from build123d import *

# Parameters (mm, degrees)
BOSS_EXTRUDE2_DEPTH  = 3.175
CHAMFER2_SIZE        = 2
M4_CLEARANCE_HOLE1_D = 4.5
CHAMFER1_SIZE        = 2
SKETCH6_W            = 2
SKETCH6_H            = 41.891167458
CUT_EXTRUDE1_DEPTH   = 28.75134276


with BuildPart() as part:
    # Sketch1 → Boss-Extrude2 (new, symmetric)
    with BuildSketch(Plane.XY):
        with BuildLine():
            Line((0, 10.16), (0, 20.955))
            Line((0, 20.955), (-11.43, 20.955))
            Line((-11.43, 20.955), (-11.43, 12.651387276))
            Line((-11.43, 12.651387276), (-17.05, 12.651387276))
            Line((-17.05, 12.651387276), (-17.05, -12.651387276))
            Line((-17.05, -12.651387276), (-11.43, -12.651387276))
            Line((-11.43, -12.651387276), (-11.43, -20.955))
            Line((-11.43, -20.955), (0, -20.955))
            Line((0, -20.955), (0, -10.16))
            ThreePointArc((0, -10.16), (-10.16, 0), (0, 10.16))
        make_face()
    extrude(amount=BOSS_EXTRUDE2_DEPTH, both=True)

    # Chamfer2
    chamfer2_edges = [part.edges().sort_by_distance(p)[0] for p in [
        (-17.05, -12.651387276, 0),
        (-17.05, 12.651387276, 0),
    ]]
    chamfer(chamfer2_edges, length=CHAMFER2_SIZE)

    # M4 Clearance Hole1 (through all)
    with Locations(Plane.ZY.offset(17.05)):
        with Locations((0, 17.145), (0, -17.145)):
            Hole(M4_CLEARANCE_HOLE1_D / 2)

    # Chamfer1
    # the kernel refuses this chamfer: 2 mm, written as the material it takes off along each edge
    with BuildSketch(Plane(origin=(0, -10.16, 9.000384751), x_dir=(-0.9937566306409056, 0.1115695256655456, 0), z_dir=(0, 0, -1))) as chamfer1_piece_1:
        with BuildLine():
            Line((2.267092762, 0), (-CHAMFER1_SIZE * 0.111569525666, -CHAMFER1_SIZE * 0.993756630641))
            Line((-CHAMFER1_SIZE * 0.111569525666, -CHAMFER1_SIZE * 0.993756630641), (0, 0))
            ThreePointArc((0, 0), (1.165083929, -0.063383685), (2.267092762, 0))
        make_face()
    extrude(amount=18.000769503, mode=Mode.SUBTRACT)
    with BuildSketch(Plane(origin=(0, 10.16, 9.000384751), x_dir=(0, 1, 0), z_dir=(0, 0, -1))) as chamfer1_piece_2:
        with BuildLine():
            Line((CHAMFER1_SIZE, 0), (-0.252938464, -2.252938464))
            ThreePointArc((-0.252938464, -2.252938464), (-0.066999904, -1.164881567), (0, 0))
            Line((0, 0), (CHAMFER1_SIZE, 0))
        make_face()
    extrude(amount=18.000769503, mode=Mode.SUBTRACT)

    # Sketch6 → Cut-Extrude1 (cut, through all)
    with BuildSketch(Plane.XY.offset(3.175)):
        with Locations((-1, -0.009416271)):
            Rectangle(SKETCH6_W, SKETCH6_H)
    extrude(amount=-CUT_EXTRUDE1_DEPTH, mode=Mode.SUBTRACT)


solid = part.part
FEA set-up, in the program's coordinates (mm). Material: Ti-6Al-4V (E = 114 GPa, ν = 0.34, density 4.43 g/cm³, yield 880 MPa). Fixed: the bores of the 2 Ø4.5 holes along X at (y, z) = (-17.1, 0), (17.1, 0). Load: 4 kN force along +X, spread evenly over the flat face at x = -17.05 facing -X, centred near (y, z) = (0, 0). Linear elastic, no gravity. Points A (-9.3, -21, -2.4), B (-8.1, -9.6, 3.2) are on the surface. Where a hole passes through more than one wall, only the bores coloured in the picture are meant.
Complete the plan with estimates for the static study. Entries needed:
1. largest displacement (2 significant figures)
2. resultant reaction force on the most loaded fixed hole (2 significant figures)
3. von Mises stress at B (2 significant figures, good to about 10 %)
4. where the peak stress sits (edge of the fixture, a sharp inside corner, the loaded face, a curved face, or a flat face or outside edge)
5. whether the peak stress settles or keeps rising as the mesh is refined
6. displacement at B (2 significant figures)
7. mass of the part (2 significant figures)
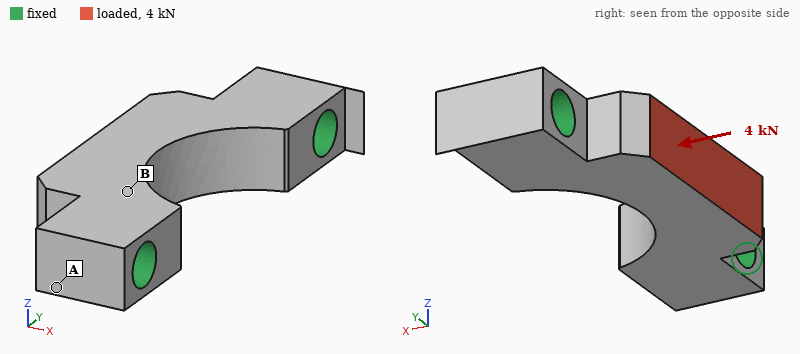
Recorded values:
14 µm
2.5 kN
51 MPa
edge of the fixture
keeps rising
5.8 µm
10 g
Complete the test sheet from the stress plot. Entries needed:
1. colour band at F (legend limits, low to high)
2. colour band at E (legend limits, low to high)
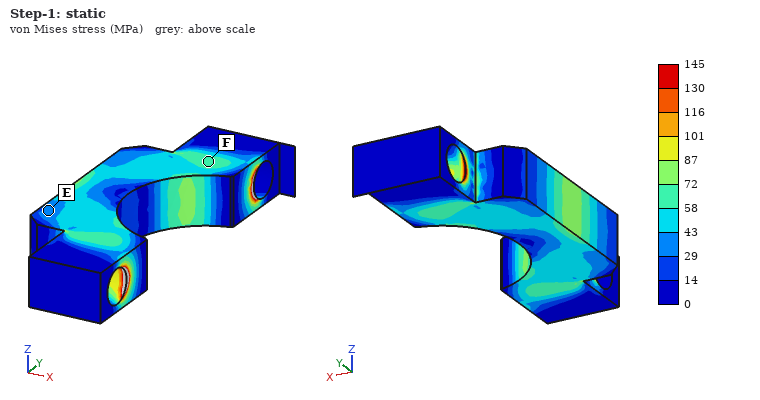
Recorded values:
58 to 72 MPa
29 to 43 MPa
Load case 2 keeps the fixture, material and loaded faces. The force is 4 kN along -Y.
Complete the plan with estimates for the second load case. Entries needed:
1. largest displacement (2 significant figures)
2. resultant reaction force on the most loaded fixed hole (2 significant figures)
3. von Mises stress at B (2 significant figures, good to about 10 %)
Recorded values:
10 µm
2.4 kN
34 MPa
